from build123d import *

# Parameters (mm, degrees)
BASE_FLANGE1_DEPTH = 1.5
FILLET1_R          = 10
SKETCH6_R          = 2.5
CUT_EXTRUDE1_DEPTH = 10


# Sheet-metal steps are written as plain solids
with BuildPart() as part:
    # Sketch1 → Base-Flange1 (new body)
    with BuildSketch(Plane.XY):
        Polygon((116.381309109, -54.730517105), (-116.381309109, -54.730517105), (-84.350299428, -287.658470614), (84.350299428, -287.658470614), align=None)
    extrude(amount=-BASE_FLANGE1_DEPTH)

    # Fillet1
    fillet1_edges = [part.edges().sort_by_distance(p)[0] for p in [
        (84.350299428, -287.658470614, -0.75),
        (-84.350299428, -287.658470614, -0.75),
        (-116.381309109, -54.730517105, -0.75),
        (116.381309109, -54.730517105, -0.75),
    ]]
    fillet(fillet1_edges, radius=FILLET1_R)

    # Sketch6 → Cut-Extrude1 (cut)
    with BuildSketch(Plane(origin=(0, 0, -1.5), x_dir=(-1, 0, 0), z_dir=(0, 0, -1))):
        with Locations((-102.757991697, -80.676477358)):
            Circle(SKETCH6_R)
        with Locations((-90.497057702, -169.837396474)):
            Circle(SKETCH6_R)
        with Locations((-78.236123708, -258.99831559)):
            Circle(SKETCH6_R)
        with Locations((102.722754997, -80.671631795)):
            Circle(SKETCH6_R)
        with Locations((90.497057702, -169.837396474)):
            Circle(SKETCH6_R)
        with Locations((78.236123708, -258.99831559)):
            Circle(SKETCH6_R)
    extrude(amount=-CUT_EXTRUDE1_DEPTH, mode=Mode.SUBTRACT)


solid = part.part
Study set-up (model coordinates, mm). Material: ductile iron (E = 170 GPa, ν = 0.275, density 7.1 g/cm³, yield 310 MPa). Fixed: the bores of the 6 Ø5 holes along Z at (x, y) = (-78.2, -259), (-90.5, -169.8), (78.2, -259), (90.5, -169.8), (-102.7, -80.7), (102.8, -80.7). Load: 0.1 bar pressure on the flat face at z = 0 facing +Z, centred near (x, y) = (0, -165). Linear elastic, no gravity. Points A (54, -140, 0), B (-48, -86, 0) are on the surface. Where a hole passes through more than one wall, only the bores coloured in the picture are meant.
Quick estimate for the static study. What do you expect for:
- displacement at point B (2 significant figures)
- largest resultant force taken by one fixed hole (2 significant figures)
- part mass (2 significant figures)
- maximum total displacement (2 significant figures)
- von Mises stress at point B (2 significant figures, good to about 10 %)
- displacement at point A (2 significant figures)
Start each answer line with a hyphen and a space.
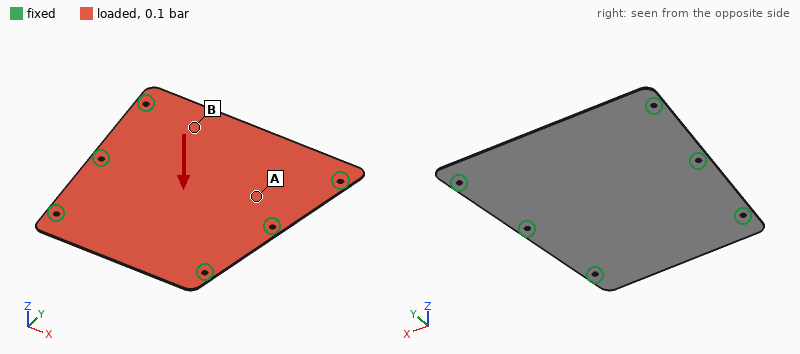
- 0.68 mm
- 91 N
- 500 g
- 1.2 mm
- 22 MPa
- 0.47 mm
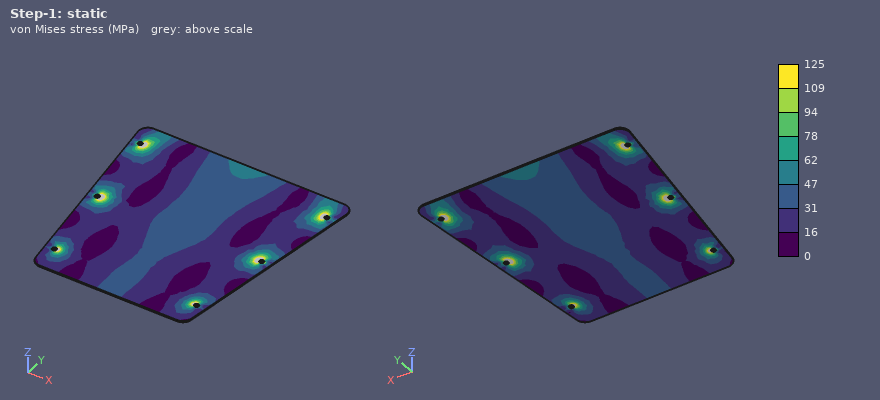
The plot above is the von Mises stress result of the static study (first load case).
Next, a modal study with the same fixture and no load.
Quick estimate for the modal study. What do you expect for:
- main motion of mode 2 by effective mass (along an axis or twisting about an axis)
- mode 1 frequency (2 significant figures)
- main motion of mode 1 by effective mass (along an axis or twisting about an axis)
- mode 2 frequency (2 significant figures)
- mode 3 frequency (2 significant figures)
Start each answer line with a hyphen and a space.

- along Z
- 180 Hz
- along Z
- 260 Hz
- 360 Hz
